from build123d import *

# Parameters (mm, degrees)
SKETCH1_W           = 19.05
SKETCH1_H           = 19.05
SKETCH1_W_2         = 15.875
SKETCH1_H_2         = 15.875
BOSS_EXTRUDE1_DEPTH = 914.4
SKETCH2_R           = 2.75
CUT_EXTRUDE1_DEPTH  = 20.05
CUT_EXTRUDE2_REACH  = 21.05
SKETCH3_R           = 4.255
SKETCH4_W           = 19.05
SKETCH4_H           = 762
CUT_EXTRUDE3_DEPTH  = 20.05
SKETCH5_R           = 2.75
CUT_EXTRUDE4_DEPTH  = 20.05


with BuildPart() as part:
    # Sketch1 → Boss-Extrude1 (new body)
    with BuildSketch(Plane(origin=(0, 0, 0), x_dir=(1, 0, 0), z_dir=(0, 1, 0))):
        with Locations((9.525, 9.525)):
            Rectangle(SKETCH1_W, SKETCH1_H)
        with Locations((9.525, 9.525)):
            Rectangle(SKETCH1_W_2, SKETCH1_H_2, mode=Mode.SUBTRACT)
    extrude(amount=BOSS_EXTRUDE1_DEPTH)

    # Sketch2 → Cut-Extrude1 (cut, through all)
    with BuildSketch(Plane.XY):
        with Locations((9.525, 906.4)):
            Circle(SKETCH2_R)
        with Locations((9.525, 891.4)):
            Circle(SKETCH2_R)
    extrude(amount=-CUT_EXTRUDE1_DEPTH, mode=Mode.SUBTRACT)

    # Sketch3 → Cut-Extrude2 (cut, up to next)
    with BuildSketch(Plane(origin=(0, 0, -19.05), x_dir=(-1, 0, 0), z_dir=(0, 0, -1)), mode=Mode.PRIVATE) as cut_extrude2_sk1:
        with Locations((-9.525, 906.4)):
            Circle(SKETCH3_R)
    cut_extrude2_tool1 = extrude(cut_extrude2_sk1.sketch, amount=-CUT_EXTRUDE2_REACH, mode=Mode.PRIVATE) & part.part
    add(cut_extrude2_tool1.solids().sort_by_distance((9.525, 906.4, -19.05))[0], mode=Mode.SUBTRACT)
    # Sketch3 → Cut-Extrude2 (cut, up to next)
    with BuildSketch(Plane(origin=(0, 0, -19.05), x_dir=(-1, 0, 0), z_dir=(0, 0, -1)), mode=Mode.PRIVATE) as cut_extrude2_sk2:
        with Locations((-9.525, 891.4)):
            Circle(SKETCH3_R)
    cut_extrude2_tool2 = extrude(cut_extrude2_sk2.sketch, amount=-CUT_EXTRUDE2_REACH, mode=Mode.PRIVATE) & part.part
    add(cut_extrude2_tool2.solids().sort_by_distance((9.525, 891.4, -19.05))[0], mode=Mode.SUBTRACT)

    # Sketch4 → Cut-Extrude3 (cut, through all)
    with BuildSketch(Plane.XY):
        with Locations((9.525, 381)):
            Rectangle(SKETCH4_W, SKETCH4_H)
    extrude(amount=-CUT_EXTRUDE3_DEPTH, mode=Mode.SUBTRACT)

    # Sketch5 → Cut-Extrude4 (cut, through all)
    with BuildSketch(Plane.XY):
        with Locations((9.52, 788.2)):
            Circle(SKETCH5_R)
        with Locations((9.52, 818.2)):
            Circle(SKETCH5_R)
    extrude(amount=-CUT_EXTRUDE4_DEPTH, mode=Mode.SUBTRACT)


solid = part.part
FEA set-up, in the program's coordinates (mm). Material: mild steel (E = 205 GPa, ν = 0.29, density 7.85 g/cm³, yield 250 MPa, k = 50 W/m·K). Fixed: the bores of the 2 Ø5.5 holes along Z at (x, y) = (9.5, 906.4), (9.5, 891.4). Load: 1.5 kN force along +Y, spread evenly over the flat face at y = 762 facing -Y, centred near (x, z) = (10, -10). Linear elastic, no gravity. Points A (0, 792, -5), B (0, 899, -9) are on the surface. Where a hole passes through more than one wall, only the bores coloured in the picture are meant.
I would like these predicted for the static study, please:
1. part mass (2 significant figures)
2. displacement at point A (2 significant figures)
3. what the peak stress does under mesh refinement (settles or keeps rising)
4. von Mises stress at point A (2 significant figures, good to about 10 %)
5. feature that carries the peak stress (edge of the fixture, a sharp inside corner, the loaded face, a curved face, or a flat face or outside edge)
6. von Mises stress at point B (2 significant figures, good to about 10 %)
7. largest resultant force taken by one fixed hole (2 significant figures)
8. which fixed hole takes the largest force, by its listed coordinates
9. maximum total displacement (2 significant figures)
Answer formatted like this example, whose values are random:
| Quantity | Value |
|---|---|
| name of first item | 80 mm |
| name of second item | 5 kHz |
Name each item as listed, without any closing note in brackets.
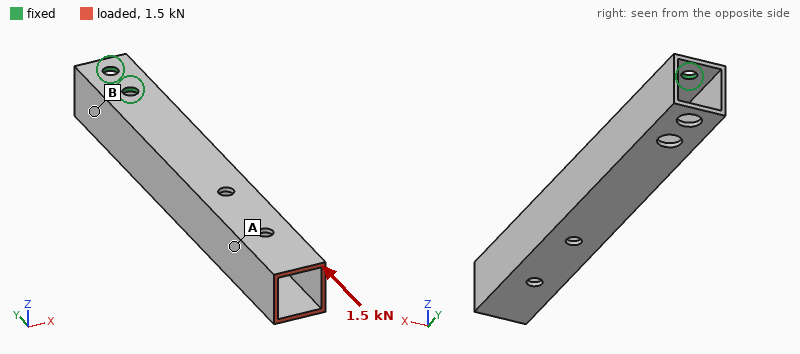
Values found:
| Quantity | Value |
|---|---|
| part mass | 130 g |
| displacement at point A | 0.23 mm |
| what the peak stress does under mesh refinement | keeps rising |
| von Mises stress at point A | 14 MPa |
| feature that carries the peak stress | edge of the fixture |
| von Mises stress at point B | 35 MPa |
| largest resultant force taken by one fixed hole | 1.2 kN |
| which fixed hole takes the largest force, by its listed coordinates | (9.5, 891.4) |
| maximum total displacement | 0.29 mm |
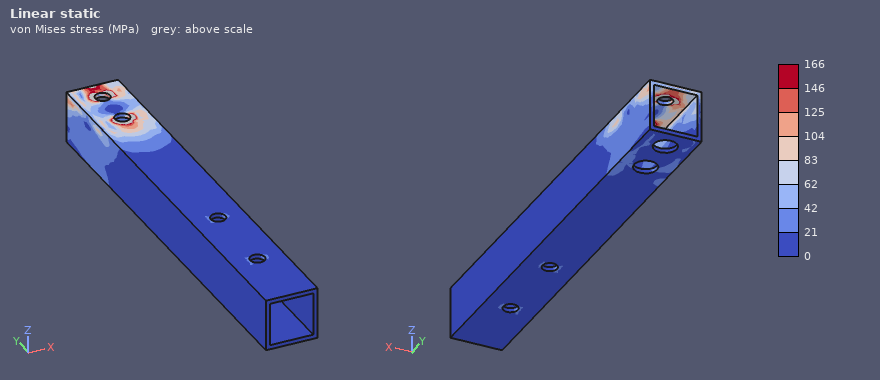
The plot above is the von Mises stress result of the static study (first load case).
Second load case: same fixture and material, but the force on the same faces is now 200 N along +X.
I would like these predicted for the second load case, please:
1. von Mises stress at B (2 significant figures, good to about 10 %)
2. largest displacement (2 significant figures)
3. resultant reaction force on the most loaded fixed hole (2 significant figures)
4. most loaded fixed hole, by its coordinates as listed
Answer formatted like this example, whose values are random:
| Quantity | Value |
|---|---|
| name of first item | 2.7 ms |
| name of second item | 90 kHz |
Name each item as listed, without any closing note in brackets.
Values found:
| Quantity | Value |
|---|---|
| von Mises stress at B | 38 MPa |
| largest displacement | 0.27 mm |
| resultant reaction force on the most loaded fixed hole | 1.2 kN |
| most loaded fixed hole, by its coordinates as listed | (9.5, 891.4) |
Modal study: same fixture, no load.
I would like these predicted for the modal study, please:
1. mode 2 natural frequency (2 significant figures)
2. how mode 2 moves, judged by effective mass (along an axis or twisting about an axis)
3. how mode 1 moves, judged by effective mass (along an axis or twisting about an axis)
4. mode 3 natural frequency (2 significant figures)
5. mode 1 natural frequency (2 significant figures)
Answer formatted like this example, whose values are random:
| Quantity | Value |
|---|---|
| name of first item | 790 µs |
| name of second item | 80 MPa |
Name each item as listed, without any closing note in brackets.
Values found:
| Quantity | Value |
|---|---|
| mode 2 natural frequency | 750 Hz |
| how mode 2 moves, judged by effective mass | along X |
| how mode 1 moves, judged by effective mass | along Z |
| mode 3 natural frequency | 1500 Hz |
| mode 1 natural frequency | 430 Hz |
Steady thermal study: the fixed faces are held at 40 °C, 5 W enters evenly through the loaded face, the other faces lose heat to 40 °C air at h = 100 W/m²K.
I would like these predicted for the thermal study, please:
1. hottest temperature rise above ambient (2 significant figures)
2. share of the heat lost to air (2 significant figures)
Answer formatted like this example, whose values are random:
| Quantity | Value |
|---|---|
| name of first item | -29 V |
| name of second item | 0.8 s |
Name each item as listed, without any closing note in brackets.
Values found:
| Quantity | Value |
|---|---|
| hottest temperature rise above ambient | 18 K |
| share of the heat lost to air | 100 % |
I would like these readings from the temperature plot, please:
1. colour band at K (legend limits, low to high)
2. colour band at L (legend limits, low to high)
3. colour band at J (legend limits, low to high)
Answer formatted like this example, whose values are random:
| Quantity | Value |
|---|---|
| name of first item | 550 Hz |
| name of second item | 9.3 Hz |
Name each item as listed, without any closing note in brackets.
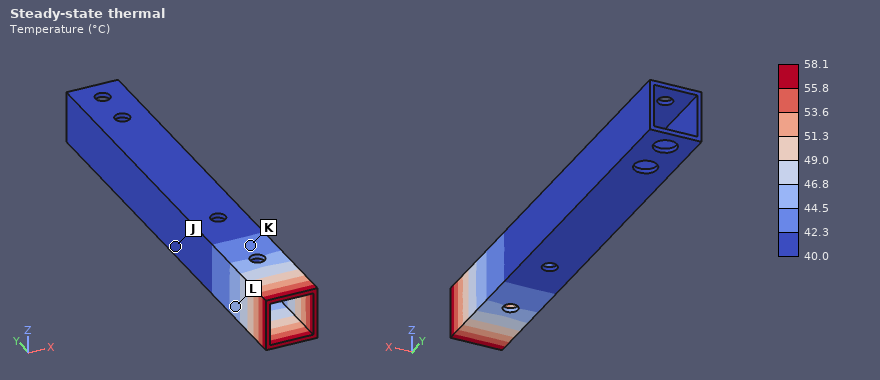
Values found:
| Quantity | Value |
|---|---|
| colour band at K | 42.3 to 44.5 °C |
| colour band at L | 44.5 to 46.8 °C |
| colour band at J | 40.0 to 42.3 °C |
